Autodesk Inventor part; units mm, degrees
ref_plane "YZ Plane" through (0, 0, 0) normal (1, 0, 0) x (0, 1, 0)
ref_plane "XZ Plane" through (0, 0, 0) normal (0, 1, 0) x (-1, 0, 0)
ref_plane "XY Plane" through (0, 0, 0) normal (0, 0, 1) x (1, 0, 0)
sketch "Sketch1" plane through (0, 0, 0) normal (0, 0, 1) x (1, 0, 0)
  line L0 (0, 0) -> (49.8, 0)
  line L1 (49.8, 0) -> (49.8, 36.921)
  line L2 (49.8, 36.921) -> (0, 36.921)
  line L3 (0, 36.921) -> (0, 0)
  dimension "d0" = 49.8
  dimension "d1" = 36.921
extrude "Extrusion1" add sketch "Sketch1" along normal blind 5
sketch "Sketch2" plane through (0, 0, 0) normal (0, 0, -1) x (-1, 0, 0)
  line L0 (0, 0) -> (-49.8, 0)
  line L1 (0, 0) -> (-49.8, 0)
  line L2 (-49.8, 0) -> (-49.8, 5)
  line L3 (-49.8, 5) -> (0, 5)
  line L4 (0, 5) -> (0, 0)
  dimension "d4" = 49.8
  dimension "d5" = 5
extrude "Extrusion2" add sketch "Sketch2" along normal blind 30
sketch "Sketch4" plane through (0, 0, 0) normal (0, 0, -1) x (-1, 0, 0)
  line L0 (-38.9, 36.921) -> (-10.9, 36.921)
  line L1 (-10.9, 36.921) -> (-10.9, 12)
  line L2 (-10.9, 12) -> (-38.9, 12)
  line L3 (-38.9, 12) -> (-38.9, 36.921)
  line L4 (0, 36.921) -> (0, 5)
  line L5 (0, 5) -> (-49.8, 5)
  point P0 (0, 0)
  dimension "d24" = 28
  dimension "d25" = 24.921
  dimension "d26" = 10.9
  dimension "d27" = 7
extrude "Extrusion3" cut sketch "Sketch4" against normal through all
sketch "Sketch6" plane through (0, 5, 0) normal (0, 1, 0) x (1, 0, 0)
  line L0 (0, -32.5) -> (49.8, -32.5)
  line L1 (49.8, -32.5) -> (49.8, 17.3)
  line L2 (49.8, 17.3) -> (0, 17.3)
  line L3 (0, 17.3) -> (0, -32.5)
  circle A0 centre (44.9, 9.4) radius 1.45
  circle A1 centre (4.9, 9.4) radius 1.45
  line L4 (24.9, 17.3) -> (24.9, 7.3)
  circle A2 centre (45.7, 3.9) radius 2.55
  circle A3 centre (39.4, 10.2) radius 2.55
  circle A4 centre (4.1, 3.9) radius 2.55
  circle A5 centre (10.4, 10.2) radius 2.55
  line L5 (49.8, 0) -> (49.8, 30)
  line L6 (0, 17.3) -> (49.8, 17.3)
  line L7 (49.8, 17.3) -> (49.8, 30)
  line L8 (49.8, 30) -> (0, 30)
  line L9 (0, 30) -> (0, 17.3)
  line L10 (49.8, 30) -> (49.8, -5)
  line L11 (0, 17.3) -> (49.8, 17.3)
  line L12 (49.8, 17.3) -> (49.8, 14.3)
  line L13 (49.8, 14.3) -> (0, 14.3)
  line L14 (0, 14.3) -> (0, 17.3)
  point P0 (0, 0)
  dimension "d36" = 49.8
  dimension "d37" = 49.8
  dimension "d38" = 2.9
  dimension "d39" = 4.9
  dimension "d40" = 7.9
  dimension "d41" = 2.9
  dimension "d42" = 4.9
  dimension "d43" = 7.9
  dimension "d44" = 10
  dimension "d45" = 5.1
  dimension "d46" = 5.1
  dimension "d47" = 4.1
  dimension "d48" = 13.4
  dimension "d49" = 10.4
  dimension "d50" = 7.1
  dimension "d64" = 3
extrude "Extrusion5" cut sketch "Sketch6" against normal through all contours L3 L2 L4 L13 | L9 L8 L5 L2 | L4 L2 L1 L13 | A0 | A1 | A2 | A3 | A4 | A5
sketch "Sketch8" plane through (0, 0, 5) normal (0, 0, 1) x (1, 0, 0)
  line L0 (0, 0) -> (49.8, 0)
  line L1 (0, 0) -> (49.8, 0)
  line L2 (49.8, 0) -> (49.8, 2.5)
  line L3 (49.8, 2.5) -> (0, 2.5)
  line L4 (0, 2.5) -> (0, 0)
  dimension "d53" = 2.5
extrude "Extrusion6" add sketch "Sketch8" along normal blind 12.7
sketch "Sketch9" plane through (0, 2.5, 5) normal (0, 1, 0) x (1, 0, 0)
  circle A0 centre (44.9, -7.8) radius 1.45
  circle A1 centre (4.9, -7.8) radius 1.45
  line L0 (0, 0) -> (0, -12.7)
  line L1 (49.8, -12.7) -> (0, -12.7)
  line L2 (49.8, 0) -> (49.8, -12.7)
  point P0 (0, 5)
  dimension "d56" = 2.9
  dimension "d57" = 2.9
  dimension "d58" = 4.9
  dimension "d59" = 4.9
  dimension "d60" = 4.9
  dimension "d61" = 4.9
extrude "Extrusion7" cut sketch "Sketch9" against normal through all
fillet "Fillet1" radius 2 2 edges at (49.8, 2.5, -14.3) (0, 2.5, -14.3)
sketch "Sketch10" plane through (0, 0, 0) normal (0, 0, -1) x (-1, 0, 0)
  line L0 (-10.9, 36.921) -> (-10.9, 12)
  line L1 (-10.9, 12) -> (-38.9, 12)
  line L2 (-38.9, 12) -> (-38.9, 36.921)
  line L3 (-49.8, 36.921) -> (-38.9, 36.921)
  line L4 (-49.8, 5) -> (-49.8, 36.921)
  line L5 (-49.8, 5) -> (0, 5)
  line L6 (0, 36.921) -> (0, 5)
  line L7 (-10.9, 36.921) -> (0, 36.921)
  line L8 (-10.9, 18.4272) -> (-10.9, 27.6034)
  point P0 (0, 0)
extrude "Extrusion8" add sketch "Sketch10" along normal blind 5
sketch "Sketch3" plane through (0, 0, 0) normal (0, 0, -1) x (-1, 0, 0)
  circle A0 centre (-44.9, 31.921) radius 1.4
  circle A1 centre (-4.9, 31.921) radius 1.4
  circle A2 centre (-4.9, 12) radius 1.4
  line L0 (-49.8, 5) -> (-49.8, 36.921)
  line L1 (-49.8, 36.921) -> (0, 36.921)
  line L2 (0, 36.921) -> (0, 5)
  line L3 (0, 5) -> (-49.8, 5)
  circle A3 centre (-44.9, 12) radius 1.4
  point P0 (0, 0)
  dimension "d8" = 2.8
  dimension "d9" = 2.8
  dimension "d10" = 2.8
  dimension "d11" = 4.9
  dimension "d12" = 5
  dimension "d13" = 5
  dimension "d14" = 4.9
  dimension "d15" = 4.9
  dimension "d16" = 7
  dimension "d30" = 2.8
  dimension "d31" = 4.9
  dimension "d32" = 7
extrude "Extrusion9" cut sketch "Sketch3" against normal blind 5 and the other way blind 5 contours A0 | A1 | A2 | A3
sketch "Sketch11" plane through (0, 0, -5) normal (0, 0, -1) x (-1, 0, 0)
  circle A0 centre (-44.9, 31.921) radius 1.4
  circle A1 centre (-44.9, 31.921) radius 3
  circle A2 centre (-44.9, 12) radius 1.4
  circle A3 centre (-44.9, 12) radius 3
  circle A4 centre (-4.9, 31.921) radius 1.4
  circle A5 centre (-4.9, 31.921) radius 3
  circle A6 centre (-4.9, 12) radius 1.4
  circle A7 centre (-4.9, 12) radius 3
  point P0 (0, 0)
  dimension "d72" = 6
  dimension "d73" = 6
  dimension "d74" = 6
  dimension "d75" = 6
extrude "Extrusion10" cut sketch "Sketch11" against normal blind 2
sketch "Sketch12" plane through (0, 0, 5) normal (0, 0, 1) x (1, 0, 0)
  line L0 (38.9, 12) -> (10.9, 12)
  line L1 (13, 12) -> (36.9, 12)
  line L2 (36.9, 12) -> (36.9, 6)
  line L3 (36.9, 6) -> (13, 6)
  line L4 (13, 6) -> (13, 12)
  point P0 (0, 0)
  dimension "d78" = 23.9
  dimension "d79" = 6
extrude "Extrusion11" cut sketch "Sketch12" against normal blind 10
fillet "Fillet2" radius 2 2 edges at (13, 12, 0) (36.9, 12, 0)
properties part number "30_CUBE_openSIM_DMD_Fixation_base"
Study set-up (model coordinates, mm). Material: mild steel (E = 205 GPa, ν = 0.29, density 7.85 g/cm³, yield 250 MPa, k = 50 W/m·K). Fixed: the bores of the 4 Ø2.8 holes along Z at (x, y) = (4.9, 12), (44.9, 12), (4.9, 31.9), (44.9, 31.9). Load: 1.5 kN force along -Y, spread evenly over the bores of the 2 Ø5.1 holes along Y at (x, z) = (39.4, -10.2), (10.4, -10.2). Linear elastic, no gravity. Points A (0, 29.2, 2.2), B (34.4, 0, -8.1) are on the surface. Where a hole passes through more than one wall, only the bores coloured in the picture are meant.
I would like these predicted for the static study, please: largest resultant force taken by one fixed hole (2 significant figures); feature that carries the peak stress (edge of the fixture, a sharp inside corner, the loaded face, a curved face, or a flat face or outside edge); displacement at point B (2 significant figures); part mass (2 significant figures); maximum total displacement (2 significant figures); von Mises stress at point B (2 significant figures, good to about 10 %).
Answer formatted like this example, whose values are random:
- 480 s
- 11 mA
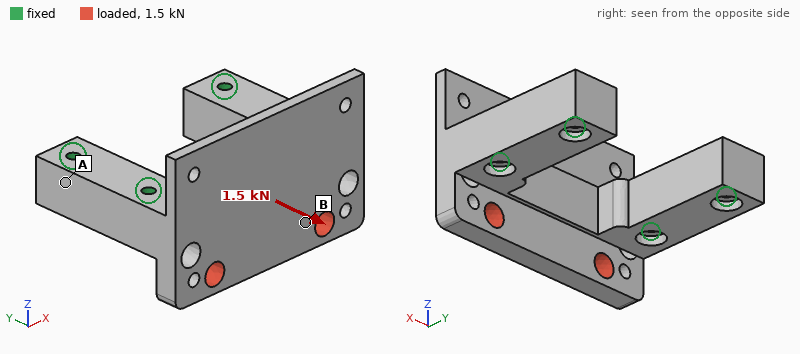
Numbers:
- 620 N
- a curved face
- 10 µm
- 100 g
- 18 µm
- 34 MPa
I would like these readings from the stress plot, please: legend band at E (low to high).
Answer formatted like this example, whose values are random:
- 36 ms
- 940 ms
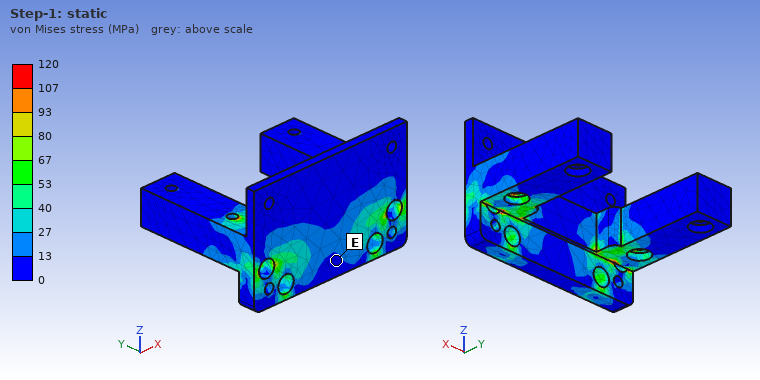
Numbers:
- 0 to 13 MPa
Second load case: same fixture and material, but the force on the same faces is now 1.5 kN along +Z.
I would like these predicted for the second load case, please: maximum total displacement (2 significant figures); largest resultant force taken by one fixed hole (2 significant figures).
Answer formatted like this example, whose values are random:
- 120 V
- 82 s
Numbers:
- 7.3 µm
- 860 N
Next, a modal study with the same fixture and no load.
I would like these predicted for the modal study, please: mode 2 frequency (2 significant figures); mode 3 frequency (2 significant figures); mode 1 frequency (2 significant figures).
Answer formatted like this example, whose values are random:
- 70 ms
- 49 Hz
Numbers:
- 12 kHz
- 13 kHz
- 8600 Hz
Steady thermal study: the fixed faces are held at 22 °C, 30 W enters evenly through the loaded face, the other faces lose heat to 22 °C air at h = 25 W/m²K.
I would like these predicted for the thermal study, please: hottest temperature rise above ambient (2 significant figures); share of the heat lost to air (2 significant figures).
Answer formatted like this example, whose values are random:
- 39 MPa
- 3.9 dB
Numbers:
- 67 K
- 11 %
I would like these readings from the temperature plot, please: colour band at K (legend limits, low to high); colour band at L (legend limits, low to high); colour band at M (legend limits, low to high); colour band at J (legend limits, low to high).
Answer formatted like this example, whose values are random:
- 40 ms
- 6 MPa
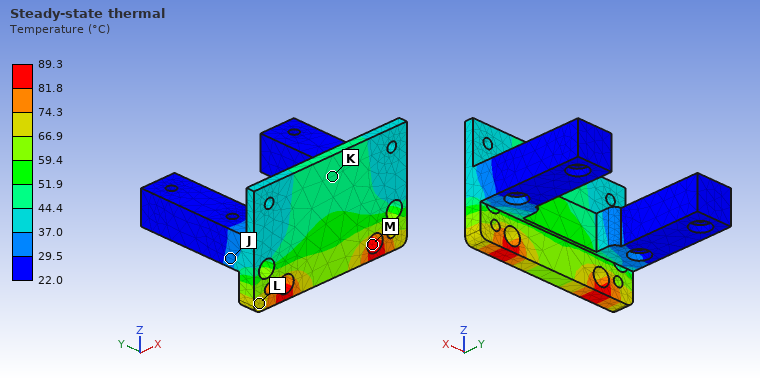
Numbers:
- 44.4 to 51.9 °C
- 66.9 to 74.3 °C
- 81.8 to 89.3 °C
- 29.5 to 37.0 °C
